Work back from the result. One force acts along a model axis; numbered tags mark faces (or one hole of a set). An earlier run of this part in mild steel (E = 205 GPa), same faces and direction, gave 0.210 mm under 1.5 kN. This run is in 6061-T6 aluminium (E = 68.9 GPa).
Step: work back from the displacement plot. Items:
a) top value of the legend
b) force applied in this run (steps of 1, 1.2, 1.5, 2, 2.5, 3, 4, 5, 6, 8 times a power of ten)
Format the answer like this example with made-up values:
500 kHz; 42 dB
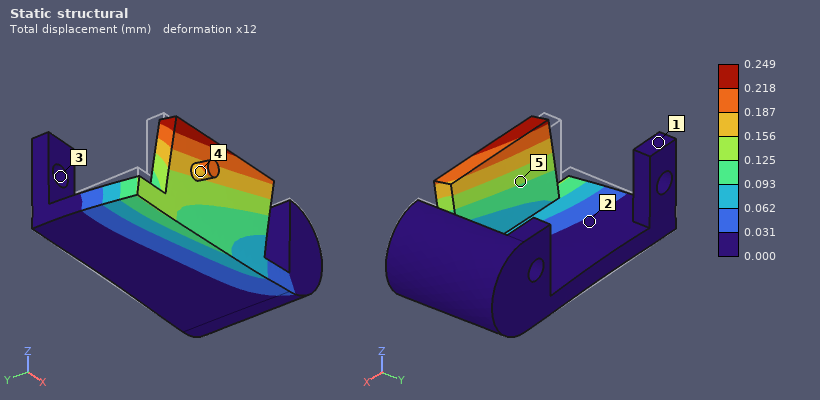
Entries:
0.249 mm; 600 N
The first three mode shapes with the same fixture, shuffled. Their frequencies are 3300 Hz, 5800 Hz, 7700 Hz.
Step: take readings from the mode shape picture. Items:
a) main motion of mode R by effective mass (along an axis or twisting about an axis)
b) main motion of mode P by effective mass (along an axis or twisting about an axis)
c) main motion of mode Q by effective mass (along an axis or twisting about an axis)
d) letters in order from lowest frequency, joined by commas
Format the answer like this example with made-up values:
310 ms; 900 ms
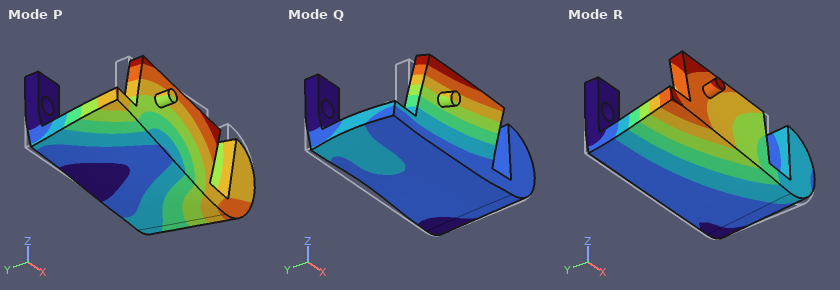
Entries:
along Z; along X; along Y; R, P, Q
